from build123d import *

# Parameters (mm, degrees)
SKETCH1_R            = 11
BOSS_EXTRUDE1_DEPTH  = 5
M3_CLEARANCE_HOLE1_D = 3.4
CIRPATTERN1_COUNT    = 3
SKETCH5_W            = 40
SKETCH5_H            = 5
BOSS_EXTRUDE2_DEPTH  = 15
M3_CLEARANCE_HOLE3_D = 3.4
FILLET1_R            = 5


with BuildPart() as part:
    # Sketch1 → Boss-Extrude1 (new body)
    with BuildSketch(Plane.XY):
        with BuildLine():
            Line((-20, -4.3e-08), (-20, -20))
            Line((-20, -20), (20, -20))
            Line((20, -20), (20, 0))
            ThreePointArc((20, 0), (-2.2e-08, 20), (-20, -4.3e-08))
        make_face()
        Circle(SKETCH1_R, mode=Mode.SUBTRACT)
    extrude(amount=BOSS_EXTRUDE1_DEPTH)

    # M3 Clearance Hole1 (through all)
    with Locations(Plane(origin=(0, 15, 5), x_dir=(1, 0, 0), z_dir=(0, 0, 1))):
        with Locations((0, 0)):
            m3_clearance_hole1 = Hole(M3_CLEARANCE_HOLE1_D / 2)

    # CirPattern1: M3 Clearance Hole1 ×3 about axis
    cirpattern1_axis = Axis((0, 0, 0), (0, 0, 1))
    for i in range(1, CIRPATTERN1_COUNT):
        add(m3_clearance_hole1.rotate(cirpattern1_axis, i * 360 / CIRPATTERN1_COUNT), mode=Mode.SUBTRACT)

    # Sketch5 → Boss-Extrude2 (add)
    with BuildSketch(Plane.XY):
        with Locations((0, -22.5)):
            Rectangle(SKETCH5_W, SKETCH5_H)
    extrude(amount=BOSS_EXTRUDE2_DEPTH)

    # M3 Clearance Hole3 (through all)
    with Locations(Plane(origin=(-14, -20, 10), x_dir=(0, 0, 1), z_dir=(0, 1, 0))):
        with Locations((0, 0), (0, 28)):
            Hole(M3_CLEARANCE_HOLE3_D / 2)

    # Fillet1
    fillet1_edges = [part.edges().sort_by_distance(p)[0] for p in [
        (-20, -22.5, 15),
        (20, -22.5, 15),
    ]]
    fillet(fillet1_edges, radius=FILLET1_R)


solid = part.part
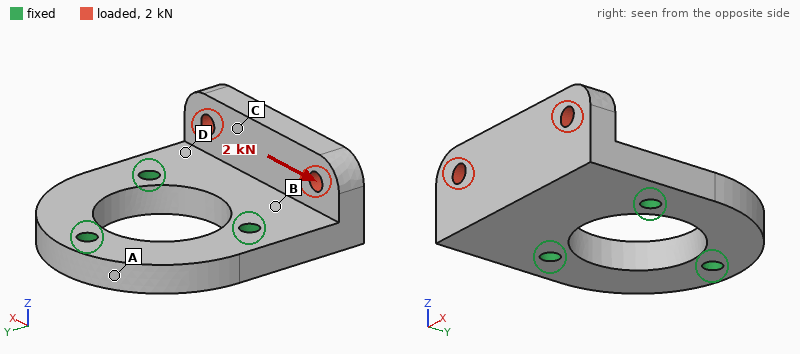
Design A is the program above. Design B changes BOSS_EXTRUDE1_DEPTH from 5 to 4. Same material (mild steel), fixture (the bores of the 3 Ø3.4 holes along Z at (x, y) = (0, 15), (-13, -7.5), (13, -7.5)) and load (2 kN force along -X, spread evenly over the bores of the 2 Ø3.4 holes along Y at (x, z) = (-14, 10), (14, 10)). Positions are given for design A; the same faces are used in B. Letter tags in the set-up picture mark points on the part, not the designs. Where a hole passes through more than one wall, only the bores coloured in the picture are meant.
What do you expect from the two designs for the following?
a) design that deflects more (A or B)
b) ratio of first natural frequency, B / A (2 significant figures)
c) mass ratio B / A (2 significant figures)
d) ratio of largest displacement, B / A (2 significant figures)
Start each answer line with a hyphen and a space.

- B
- 0.74
- 0.87
- 1.6
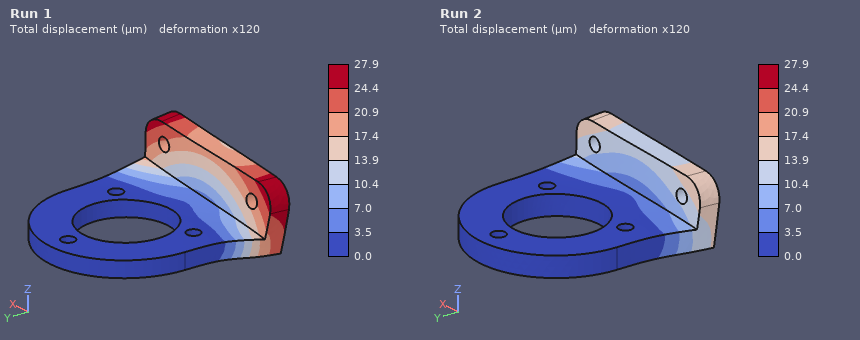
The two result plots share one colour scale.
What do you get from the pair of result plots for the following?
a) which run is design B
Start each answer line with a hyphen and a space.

- Run 1
